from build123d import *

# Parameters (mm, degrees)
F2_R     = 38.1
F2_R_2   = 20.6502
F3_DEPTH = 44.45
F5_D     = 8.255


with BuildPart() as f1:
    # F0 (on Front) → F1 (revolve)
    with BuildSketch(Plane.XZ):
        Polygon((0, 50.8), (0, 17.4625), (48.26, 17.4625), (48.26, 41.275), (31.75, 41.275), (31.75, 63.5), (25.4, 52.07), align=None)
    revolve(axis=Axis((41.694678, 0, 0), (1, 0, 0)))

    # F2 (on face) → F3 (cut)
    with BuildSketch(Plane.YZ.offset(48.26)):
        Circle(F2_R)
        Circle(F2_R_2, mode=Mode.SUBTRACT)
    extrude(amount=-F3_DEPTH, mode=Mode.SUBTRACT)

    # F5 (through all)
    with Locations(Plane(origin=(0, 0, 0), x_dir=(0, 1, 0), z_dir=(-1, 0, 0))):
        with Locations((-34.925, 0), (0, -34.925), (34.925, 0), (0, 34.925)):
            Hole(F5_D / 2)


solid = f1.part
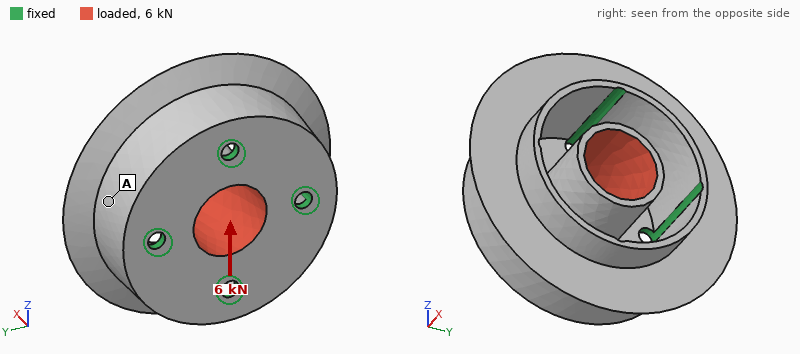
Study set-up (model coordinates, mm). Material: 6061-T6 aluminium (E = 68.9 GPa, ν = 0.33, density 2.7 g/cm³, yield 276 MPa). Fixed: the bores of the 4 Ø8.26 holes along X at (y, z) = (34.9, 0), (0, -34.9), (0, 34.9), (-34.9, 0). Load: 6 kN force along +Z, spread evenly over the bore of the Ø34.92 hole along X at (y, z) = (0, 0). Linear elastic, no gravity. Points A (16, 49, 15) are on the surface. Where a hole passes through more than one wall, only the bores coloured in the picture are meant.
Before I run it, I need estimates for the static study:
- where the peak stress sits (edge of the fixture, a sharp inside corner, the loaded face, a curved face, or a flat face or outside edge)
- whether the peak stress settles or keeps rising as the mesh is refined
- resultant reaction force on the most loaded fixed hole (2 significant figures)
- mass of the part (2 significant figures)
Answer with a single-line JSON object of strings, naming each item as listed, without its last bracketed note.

{"where the peak stress sits": "edge of the fixture", "whether the peak stress settles or keeps rising as the mesh is refined": "keeps rising", "resultant reaction force on the most loaded fixed hole": "2.9 kN", "mass of the part": "470 g"}
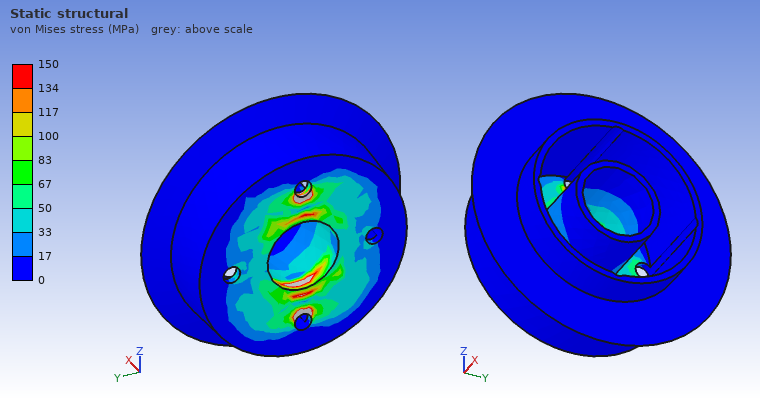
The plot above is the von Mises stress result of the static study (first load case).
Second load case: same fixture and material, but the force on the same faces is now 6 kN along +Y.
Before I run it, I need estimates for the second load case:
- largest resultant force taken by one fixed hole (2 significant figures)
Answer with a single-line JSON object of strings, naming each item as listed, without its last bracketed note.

{"largest resultant force taken by one fixed hole": "2.9 kN"}
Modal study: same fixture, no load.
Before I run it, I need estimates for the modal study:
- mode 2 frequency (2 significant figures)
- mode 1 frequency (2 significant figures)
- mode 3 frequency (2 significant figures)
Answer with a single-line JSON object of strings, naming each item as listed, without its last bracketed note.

{"mode 2 frequency": "4400 Hz", "mode 1 frequency": "4300 Hz", "mode 3 frequency": "6700 Hz"}
